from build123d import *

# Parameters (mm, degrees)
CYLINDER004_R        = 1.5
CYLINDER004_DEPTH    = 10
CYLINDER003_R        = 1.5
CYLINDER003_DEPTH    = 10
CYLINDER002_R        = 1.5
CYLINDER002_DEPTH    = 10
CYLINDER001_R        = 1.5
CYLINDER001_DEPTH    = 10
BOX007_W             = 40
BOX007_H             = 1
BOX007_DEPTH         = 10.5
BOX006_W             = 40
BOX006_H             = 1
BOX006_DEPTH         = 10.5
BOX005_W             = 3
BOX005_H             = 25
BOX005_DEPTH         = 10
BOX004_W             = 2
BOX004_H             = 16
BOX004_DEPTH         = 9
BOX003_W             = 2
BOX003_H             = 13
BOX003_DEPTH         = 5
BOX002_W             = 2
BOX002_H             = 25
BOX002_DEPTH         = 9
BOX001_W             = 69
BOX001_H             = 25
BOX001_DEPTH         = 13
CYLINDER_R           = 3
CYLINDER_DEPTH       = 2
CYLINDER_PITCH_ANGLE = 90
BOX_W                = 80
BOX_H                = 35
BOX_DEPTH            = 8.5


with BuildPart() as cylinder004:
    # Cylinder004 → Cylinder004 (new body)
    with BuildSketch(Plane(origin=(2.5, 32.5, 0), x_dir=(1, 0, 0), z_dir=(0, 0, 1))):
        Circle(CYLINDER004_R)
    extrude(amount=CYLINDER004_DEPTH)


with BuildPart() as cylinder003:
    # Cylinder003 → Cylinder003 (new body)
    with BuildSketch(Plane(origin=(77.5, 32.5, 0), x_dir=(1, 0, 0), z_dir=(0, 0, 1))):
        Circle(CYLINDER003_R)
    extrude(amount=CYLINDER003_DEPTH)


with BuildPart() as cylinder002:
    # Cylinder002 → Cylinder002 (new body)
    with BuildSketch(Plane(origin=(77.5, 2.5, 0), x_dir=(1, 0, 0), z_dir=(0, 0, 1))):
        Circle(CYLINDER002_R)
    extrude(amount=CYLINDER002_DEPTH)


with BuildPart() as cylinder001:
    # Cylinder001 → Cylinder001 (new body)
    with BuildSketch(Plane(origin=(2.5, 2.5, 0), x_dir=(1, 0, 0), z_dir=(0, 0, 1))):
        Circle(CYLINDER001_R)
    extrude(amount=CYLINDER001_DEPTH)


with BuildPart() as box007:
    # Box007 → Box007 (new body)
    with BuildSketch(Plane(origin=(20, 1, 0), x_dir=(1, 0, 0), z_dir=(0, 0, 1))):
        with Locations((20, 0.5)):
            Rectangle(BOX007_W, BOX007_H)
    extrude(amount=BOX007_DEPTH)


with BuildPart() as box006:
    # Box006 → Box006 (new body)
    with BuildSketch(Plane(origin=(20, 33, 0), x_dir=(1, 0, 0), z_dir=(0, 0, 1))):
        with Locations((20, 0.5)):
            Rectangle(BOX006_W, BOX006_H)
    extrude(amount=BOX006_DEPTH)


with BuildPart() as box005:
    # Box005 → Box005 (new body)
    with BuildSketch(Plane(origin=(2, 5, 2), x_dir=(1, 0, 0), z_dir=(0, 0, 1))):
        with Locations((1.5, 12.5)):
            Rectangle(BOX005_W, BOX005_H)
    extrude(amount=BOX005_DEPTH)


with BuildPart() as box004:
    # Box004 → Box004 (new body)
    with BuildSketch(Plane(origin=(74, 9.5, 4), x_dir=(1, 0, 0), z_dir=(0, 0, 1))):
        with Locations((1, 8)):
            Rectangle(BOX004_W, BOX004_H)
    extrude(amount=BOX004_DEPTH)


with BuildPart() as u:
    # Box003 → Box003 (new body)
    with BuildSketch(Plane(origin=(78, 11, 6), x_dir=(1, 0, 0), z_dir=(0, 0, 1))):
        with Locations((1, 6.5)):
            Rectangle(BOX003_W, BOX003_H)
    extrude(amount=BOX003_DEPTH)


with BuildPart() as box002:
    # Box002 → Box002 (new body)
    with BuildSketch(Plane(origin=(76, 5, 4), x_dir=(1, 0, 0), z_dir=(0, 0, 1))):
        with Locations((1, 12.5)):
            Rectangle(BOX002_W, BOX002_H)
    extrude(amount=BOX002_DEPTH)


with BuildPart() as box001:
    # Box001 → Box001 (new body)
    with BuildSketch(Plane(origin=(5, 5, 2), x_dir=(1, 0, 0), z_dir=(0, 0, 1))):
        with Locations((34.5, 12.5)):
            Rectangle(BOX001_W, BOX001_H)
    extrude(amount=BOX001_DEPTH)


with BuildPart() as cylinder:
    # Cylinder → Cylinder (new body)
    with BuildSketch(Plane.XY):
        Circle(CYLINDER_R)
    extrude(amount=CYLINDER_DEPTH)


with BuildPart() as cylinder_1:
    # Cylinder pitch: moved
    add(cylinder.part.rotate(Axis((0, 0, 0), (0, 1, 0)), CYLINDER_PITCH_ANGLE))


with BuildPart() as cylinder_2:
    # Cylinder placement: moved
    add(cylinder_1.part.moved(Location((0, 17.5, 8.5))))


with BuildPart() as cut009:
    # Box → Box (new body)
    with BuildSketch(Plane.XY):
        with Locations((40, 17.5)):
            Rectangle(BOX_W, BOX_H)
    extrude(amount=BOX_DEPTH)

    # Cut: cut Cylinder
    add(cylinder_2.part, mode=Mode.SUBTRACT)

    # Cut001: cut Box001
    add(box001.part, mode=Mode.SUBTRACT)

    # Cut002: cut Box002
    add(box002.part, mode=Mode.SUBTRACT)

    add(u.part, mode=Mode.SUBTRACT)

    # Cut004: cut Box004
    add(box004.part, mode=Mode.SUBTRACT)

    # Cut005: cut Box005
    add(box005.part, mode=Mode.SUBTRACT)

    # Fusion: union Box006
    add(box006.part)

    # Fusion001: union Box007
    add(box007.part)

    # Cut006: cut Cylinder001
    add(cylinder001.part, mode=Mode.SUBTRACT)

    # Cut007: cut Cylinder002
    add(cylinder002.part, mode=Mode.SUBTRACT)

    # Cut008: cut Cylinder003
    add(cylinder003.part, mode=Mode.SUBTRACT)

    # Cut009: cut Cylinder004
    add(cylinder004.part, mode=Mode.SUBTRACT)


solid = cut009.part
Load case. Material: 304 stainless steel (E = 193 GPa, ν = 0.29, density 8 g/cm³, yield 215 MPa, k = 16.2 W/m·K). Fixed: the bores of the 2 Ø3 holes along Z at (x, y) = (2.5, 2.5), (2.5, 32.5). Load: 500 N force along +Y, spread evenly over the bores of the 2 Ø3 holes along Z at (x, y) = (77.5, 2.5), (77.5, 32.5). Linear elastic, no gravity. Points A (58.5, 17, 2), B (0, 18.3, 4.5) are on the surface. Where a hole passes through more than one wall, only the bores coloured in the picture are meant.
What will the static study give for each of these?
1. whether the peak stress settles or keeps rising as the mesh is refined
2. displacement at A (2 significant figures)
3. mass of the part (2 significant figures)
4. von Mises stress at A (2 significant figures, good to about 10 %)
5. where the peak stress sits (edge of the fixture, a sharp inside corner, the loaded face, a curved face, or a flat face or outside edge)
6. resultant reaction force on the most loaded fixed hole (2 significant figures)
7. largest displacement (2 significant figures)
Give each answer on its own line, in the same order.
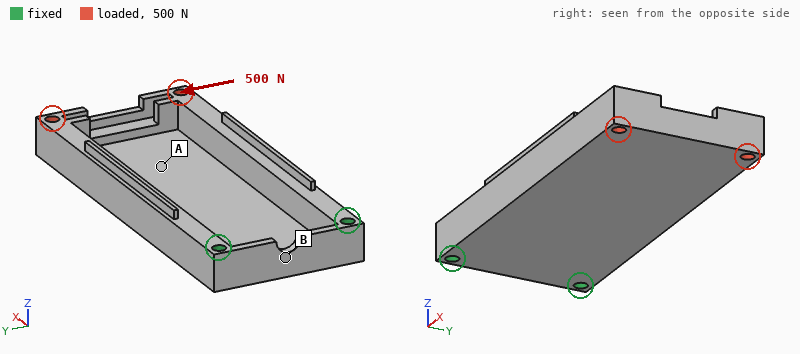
keeps rising
24 µm
92 g
32 MPa
edge of the fixture
1.2 kN
82 µm
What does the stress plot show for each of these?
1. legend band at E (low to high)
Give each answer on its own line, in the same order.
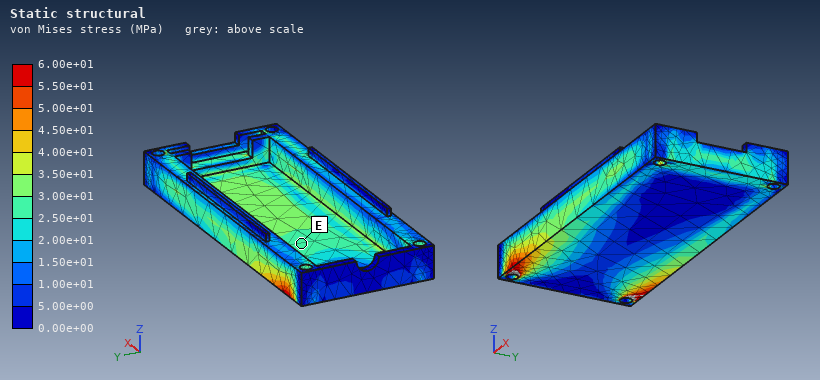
2.50e+01 to 3.00e+01 MPa
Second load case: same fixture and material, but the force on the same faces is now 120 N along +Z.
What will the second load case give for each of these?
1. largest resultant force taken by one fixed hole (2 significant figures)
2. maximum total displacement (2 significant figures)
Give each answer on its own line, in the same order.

150 N
0.11 mm
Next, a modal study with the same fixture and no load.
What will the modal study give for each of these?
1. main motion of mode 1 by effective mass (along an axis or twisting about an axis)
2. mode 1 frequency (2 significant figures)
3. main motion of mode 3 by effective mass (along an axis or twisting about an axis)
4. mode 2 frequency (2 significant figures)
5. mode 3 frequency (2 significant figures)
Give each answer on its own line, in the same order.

along Z
1000 Hz
along Y
2000 Hz
4500 Hz
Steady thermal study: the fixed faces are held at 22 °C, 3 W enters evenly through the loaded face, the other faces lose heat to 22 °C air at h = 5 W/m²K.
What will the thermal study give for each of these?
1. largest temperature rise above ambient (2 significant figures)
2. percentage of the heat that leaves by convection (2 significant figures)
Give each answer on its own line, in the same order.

73 K
47 %
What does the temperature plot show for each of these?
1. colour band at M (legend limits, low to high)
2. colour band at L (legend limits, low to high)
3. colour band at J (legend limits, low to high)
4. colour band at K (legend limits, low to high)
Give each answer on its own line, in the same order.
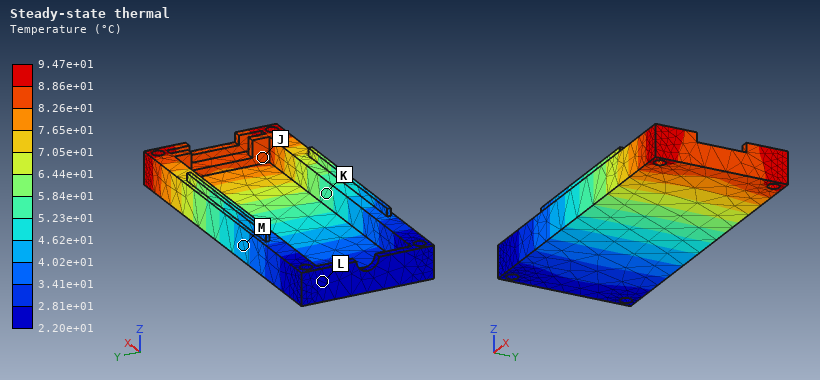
4.02e+01 to 4.62e+01 °C
2.20e+01 to 2.81e+01 °C
8.26e+01 to 8.86e+01 °C
5.23e+01 to 5.84e+01 °C
